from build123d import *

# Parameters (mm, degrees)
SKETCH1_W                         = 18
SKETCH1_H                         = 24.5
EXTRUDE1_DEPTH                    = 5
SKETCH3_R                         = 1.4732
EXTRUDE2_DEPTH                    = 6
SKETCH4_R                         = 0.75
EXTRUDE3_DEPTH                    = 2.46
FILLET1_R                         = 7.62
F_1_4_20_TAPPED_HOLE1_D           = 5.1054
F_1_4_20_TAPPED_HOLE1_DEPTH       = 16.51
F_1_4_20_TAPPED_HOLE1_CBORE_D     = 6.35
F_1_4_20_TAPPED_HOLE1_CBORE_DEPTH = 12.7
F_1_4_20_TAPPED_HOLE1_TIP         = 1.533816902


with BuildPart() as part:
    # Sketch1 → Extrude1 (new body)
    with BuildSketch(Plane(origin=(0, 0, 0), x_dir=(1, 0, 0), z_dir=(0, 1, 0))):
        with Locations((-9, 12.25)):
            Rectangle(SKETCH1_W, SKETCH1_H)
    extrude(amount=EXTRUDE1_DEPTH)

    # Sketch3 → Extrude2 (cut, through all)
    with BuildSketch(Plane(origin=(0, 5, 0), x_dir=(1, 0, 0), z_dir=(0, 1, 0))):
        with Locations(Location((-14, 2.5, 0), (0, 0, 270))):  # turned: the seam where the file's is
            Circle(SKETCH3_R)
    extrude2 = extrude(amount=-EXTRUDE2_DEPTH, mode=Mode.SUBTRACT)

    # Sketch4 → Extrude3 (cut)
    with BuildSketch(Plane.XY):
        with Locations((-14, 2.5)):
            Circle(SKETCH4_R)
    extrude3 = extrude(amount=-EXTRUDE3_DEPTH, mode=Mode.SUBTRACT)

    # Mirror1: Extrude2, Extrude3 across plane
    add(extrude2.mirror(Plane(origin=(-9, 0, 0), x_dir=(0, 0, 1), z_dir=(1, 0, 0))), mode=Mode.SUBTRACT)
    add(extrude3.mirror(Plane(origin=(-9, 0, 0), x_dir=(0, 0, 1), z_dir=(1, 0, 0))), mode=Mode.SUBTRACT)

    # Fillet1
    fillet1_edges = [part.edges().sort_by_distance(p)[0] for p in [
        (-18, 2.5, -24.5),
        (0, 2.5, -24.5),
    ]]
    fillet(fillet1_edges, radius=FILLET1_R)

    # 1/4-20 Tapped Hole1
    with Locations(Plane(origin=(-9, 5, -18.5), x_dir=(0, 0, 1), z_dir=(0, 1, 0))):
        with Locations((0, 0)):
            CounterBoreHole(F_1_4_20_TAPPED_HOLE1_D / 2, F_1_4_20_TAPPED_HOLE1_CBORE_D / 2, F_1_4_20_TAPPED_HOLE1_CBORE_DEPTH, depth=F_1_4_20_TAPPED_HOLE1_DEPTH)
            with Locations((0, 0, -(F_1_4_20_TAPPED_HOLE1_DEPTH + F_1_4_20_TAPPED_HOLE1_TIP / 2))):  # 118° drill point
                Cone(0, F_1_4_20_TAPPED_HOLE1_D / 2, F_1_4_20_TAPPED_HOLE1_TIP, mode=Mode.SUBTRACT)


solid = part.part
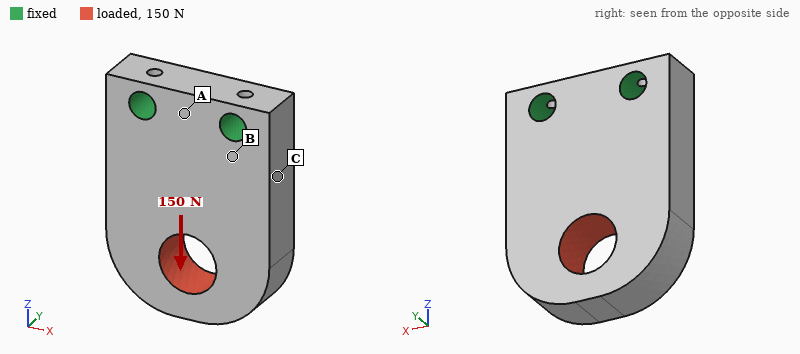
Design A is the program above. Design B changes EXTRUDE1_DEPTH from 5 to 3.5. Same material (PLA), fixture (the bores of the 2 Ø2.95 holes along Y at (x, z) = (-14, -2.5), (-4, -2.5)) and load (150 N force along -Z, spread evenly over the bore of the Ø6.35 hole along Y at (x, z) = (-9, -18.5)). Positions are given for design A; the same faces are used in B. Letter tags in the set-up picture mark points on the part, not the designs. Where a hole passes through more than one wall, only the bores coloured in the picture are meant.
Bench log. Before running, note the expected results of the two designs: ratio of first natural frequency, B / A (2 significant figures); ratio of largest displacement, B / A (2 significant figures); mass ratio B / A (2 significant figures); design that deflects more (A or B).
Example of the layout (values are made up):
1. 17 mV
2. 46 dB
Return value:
1. 0.73
2. 1.4
3. 0.70
4. B
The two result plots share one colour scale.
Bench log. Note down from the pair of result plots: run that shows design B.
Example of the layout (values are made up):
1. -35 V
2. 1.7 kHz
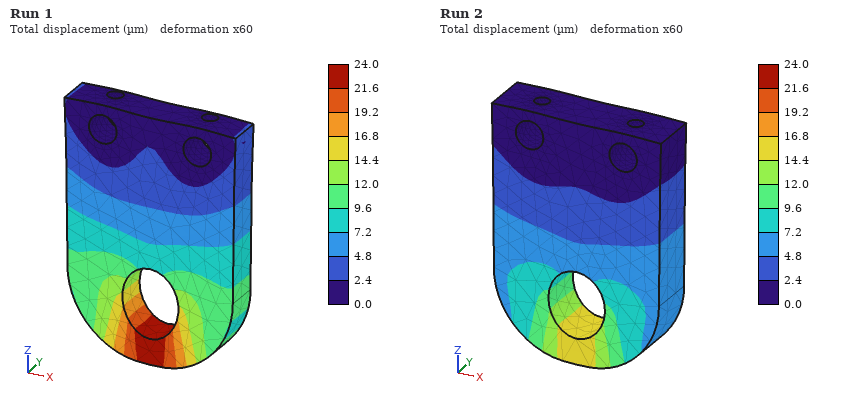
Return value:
1. Run 1
